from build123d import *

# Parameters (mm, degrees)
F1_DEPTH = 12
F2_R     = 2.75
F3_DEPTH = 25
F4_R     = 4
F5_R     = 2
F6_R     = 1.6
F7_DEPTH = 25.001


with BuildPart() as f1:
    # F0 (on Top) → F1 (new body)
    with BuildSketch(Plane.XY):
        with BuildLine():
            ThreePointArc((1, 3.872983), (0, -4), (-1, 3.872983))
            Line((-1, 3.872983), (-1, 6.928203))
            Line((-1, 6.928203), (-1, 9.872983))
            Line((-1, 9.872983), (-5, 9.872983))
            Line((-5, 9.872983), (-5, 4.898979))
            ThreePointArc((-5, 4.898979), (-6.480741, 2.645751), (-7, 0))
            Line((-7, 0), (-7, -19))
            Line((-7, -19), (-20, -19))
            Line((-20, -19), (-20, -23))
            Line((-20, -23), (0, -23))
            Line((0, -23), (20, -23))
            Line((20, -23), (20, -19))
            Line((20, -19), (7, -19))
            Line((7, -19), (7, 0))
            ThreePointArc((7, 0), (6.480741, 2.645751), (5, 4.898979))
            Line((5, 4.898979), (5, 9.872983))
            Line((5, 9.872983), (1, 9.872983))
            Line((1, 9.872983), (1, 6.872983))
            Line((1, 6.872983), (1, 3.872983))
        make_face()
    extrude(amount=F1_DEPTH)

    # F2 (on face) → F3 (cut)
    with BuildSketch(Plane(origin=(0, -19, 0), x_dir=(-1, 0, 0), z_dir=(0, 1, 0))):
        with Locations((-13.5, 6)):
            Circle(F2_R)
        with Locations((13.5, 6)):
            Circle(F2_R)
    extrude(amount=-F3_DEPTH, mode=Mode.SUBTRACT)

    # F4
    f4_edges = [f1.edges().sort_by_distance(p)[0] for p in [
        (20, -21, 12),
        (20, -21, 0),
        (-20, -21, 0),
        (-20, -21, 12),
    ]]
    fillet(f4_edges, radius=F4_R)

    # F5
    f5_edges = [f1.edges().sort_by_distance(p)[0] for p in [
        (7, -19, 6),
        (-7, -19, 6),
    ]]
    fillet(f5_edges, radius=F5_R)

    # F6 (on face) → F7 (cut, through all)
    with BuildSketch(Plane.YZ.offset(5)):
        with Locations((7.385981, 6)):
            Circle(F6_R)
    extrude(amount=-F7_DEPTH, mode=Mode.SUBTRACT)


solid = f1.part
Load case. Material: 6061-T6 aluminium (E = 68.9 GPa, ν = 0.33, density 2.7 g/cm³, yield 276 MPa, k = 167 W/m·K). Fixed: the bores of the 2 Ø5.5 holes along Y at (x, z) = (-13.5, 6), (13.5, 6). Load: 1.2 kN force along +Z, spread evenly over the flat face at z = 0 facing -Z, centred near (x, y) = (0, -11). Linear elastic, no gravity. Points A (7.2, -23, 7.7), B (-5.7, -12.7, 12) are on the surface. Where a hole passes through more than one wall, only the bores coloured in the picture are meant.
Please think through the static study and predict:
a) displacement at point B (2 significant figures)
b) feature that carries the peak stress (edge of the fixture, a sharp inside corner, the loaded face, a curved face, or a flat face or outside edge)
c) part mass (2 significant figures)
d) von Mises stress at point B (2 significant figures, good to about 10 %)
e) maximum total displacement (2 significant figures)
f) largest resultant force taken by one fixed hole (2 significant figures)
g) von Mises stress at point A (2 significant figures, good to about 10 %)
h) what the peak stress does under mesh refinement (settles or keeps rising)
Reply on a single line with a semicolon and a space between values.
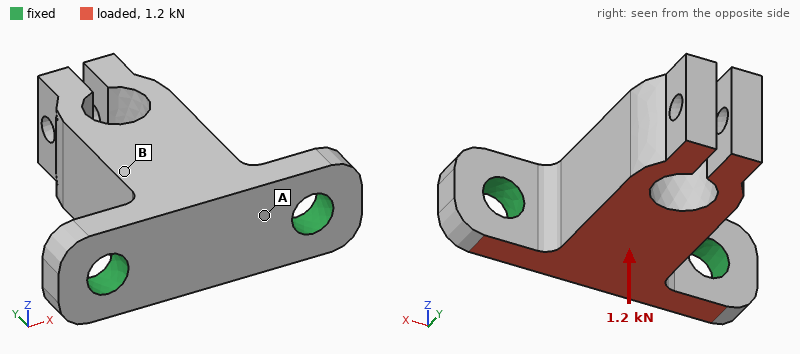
0.050 mm; edge of the fixture; 15 g; 20 MPa; 0.16 mm; 600 N; 55 MPa; keeps rising
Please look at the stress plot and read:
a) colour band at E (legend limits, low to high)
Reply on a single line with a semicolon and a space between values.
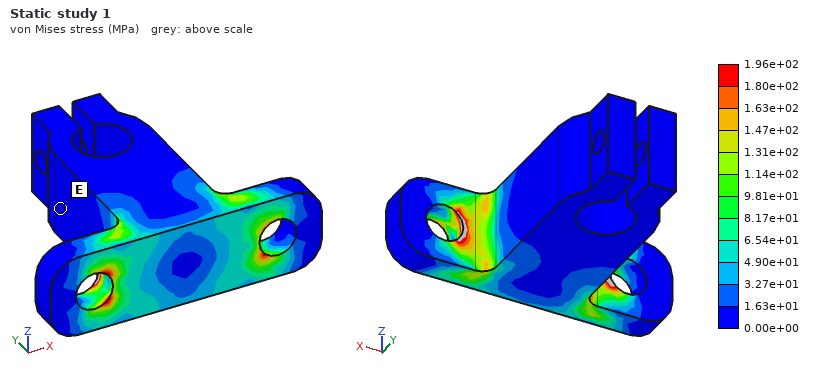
0.00e+00 to 1.63e+01 MPa
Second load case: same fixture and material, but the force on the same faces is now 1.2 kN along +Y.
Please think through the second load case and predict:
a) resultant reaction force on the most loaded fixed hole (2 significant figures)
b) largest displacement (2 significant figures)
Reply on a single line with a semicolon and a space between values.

650 N; 83 µm
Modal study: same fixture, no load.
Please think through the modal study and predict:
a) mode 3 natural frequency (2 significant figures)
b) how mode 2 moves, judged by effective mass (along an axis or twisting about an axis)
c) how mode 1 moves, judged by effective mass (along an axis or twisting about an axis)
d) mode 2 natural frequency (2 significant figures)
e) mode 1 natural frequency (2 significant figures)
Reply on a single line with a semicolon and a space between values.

12 kHz; along X; along Z; 8600 Hz; 4800 Hz
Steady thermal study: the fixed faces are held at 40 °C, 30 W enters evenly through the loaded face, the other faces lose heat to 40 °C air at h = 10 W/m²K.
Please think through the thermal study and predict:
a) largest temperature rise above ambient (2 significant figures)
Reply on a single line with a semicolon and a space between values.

24 K
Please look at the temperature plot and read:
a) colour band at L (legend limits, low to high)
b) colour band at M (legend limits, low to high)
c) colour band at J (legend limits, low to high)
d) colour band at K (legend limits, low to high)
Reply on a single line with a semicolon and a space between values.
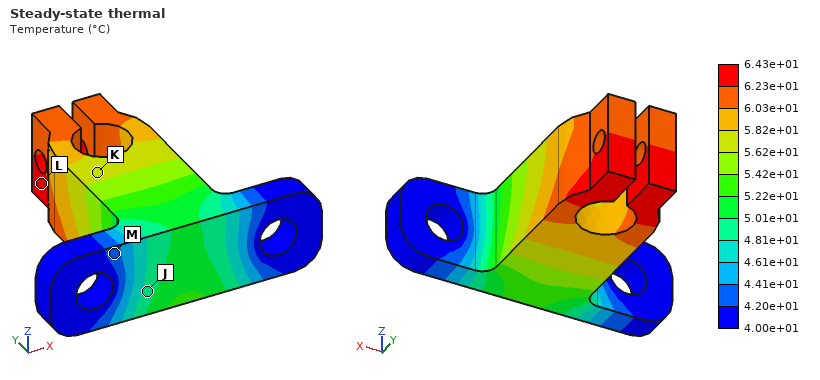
6.23e+01 to 6.43e+01 °C; 4.20e+01 to 4.41e+01 °C; 4.81e+01 to 5.01e+01 °C; 5.62e+01 to 5.82e+01 °C
